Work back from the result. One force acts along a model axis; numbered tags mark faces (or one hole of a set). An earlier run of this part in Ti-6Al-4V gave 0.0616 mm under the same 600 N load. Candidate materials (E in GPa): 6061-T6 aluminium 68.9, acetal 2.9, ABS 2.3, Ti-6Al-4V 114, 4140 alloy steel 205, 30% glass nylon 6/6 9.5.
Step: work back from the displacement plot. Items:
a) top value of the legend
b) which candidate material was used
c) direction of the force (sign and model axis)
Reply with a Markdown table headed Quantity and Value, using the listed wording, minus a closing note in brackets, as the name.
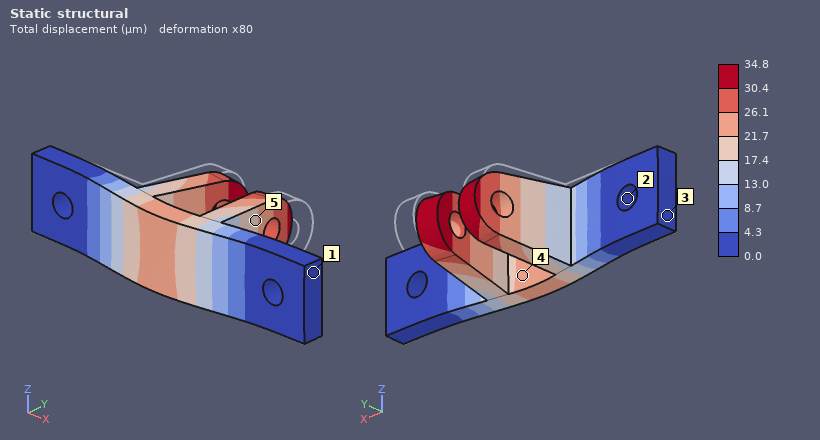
| Quantity | Value |
|---|---|
| top value of the legend | 34.8 µm |
| which candidate material was used | 4140 alloy steel |
| direction of the force | -Y |
